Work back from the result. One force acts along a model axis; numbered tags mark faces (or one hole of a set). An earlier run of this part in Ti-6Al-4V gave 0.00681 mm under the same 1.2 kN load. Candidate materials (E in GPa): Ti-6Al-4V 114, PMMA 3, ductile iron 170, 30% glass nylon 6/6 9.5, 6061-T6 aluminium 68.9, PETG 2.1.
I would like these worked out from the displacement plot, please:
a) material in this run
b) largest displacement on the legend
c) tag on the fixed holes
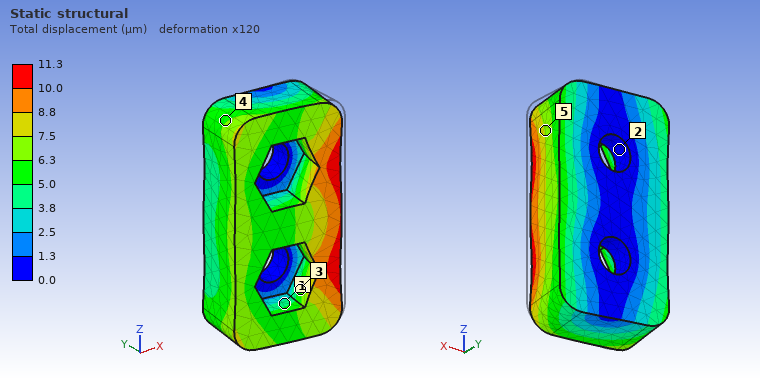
6061-T6 aluminium
11.3 µm
2
